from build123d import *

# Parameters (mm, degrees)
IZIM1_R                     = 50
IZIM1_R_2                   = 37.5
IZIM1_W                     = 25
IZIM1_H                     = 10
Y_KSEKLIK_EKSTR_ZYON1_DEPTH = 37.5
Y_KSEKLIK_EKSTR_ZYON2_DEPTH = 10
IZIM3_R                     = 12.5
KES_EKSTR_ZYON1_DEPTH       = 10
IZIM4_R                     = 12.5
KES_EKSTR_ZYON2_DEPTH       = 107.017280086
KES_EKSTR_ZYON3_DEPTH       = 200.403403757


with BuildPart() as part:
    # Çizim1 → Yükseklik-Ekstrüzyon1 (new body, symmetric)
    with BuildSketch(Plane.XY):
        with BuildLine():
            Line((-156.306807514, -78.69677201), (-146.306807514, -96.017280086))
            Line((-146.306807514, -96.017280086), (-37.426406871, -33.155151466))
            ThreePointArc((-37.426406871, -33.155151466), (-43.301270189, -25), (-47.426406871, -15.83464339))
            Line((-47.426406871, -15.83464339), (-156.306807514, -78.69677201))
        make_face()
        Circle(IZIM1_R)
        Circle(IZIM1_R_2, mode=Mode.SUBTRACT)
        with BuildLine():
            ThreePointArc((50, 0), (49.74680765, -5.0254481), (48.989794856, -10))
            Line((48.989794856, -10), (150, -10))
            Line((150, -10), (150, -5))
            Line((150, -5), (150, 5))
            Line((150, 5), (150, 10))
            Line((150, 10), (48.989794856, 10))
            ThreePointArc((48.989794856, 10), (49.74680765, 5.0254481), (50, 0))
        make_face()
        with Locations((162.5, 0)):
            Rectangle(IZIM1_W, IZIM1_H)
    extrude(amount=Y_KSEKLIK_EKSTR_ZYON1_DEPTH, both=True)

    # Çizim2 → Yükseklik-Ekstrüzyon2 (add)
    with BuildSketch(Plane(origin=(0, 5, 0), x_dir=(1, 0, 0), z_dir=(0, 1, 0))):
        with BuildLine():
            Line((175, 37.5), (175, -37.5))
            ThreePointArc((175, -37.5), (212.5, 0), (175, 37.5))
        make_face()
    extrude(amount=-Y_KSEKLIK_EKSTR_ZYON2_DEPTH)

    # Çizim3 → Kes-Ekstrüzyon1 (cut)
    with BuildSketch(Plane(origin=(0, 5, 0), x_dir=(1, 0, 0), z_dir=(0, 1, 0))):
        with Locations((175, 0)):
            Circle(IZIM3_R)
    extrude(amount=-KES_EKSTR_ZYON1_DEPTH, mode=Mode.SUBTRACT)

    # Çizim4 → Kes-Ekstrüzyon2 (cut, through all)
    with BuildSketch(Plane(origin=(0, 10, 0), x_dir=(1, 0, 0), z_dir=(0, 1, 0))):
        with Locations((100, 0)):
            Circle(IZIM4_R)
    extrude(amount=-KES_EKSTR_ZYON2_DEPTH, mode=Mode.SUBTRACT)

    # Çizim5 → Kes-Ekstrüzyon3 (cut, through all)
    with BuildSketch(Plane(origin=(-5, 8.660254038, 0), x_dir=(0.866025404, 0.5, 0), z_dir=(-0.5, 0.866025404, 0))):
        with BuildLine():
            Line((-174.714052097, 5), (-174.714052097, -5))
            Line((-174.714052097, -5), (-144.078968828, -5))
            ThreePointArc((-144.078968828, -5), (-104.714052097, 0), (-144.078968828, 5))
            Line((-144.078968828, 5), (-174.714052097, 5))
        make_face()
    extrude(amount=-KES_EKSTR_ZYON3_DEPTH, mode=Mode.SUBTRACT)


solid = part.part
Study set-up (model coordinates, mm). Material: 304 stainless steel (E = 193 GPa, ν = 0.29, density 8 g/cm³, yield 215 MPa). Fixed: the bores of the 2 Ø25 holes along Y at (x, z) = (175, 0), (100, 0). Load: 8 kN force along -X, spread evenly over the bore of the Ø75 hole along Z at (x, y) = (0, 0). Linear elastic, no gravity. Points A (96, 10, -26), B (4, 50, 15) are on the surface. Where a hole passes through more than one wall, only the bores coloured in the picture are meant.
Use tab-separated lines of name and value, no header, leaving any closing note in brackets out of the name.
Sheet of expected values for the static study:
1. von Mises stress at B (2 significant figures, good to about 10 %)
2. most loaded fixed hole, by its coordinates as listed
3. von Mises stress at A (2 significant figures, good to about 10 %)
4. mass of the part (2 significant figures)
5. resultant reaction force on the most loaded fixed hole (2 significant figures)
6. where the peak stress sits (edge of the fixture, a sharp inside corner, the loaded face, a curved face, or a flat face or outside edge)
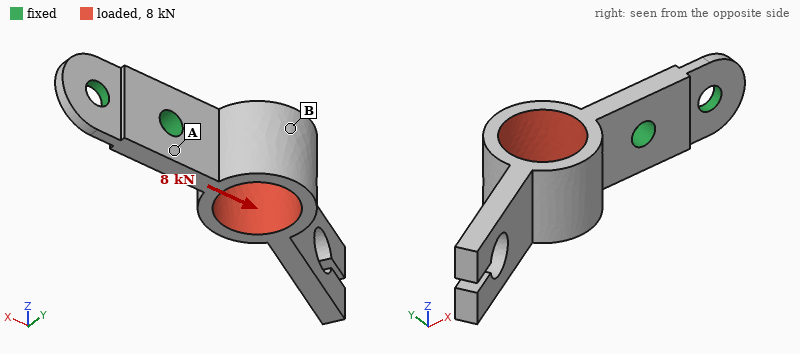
von Mises stress at B	11 MPa
most loaded fixed hole, by its coordinates as listed	(100, 0)
von Mises stress at A	2.9 MPa
mass of the part	4.7 kg
resultant reaction force on the most loaded fixed hole	7.4 kN
where the peak stress sits	the loaded face
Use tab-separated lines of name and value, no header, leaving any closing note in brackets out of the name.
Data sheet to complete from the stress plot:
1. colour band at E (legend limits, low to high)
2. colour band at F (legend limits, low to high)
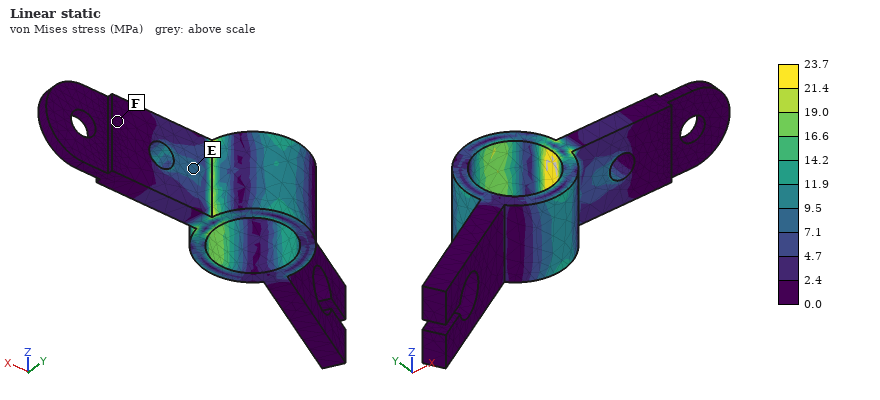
colour band at E	7.1 to 9.5 MPa
colour band at F	0.0 to 2.4 MPa
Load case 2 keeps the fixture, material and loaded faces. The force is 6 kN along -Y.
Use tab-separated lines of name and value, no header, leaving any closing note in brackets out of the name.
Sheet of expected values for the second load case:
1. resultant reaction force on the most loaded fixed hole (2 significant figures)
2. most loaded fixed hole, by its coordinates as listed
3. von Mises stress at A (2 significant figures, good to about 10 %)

resultant reaction force on the most loaded fixed hole	6.5 kN
most loaded fixed hole, by its coordinates as listed	(100, 0)
von Mises stress at A	46 MPa
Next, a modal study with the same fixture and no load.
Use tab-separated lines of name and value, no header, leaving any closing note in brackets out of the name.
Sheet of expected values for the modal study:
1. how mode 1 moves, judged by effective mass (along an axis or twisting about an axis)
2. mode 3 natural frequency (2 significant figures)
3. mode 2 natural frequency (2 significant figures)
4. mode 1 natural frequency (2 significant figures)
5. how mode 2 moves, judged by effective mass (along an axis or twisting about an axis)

how mode 1 moves, judged by effective mass	along Y
mode 3 natural frequency	1200 Hz
mode 2 natural frequency	470 Hz
mode 1 natural frequency	250 Hz
how mode 2 moves, judged by effective mass	along Z
